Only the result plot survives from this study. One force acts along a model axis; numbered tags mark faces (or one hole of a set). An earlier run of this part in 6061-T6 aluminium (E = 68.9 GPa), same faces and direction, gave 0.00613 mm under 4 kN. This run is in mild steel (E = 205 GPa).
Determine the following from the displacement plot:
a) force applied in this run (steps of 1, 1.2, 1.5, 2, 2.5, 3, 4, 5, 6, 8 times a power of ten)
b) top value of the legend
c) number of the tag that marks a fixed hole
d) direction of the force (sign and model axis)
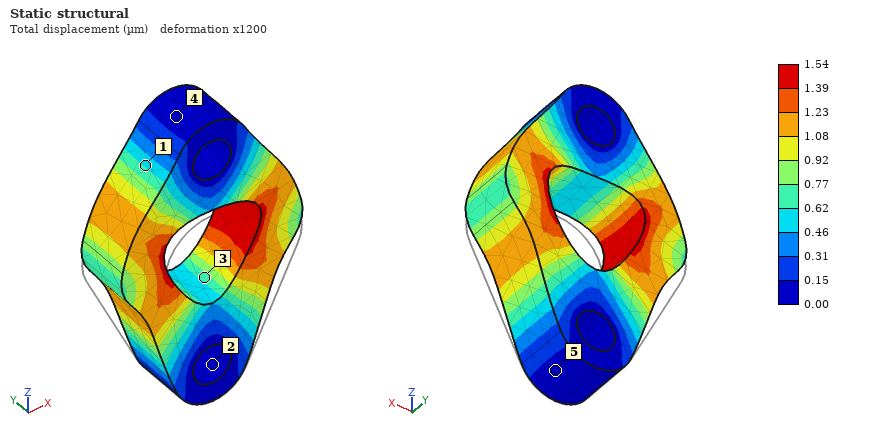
3 kN
1.54 µm
2
+Z
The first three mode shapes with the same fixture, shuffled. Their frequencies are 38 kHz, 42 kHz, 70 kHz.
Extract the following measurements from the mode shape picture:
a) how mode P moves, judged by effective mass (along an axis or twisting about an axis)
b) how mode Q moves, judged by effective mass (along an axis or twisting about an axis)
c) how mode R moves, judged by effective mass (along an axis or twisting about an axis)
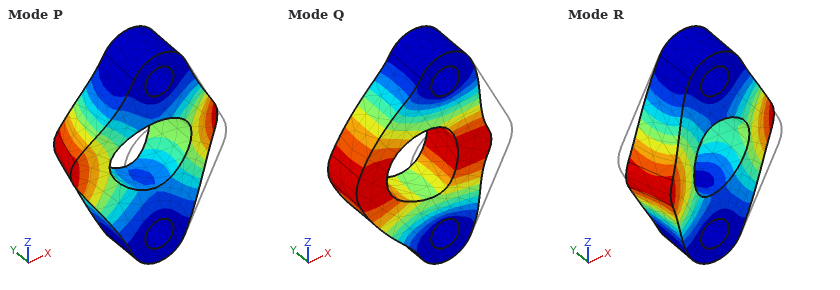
along Y
along X
twisting about Z
